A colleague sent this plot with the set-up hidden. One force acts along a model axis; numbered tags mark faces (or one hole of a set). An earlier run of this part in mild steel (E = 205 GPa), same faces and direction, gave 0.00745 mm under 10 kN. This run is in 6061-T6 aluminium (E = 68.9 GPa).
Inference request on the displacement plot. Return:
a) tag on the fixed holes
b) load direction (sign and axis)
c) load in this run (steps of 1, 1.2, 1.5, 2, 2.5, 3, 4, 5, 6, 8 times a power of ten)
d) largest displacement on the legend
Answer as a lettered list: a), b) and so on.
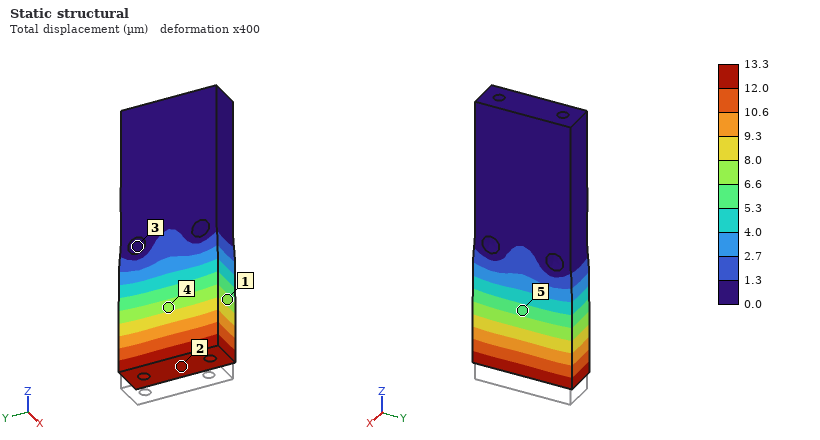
a) 3
b) +Z
c) 6 kN
d) 13.3 µm
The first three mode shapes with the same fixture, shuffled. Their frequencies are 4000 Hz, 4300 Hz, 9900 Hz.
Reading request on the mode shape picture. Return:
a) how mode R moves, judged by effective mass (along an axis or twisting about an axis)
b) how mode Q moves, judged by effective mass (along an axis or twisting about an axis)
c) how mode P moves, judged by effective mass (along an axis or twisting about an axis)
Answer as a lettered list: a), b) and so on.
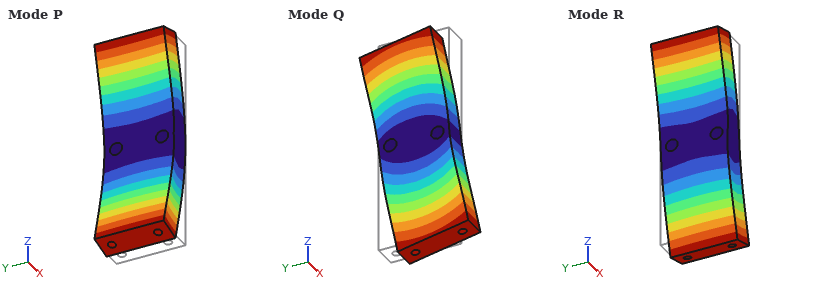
a) twisting about Y
b) twisting about X
c) along X
